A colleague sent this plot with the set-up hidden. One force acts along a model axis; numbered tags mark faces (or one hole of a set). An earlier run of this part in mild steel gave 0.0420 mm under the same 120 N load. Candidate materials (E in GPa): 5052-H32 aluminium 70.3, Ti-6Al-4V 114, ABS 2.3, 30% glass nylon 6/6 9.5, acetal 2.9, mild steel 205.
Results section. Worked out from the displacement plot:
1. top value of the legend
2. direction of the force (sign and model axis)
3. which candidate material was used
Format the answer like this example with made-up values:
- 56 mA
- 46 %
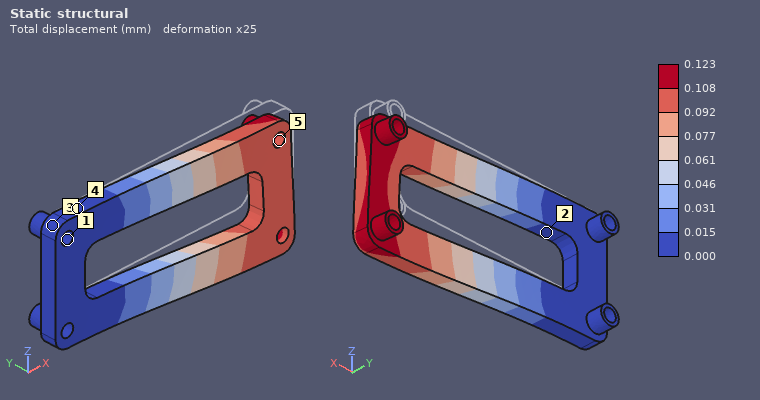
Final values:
- 0.123 mm
- -Z
- 5052-H32 aluminium
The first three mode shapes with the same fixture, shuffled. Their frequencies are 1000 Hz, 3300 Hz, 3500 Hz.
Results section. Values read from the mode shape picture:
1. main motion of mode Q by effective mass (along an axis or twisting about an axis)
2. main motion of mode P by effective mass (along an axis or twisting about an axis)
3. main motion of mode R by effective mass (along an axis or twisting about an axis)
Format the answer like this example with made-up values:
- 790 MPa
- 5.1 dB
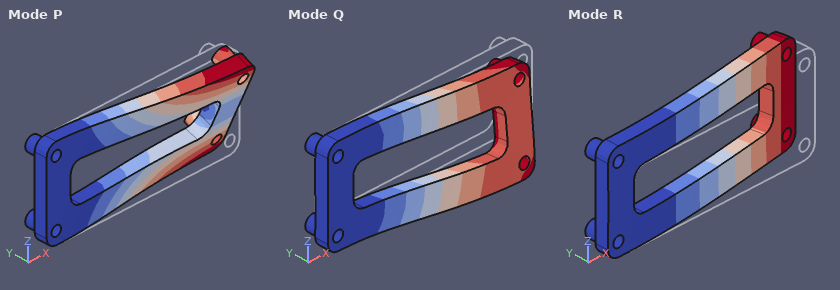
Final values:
- along Z
- twisting about X
- along Y
